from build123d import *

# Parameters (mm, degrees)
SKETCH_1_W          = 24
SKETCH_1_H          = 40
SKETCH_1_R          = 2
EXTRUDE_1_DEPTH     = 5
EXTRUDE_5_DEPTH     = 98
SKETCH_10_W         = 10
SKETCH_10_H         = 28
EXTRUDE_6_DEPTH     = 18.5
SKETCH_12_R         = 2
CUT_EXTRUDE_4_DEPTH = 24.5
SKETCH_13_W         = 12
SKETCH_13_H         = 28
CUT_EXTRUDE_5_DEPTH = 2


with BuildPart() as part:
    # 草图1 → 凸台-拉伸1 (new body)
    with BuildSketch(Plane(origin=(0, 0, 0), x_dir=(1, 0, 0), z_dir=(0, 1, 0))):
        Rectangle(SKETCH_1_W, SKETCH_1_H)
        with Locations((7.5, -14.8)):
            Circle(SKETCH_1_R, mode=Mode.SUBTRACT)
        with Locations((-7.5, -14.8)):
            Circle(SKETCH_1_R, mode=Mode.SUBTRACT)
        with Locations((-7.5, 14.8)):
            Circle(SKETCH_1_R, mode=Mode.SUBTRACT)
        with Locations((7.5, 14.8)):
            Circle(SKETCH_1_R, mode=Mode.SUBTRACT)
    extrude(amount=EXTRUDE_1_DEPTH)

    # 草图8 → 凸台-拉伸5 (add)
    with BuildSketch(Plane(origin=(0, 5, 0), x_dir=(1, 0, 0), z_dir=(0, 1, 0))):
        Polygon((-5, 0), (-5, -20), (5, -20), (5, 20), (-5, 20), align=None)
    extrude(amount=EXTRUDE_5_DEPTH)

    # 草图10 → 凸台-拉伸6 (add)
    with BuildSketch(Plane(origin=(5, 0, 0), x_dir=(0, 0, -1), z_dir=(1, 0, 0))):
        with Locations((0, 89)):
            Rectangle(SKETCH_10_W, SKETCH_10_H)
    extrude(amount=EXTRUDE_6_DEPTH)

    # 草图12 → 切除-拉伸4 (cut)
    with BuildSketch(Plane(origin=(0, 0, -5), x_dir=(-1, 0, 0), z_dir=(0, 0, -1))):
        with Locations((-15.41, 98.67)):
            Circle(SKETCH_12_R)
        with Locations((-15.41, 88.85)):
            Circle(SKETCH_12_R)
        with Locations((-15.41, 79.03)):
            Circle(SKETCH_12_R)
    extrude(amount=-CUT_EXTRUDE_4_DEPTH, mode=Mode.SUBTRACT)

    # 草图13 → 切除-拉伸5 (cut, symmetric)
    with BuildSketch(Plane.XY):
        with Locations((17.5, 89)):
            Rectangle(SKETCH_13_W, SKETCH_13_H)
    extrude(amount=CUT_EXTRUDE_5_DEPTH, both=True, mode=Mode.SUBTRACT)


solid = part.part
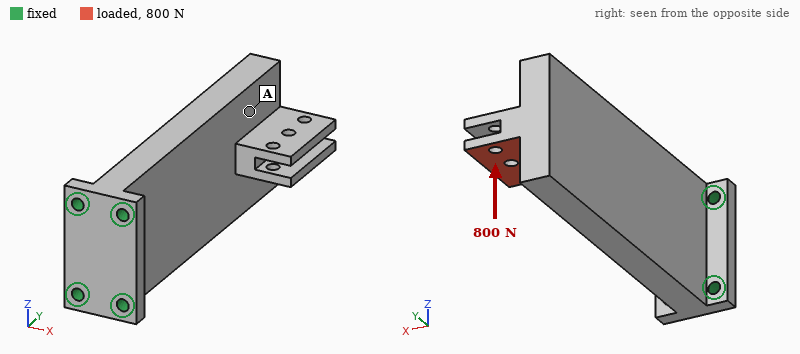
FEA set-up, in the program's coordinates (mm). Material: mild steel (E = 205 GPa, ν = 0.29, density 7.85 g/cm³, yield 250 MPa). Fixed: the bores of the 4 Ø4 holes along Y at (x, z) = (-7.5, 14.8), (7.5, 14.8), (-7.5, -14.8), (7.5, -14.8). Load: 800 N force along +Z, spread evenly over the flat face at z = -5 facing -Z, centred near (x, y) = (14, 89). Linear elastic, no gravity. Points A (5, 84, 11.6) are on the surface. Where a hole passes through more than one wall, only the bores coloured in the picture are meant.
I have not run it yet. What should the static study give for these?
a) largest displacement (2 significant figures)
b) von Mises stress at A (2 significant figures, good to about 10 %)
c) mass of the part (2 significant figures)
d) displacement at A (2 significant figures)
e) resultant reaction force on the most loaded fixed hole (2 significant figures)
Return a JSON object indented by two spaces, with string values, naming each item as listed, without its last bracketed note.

{
  "largest displacement": "70 µm",
  "von Mises stress at A": "12 MPa",
  "mass of the part": "370 g",
  "displacement at A": "28 µm",
  "resultant reaction force on the most loaded fixed hole": "1.5 kN"
}
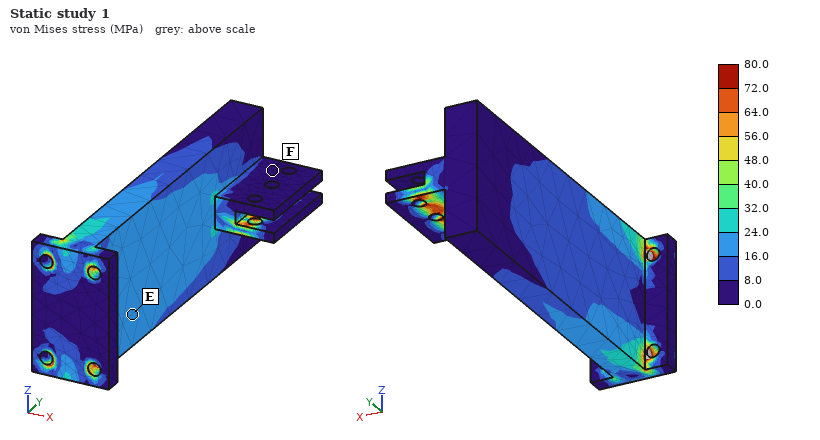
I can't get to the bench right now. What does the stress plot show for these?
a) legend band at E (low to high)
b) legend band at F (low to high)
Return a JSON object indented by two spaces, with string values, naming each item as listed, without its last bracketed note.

{
  "legend band at E": "16.0 to 24.0 MPa",
  "legend band at F": "0.0 to 8.0 MPa"
}
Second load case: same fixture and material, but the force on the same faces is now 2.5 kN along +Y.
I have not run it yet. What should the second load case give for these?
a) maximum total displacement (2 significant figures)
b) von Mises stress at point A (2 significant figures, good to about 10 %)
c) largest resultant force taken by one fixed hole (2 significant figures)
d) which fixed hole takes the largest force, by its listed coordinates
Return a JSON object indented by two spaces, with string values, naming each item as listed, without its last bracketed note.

{
  "maximum total displacement": "0.29 mm",
  "von Mises stress at point A": "26 MPa",
  "largest resultant force taken by one fixed hole": "2.2 kN",
  "which fixed hole takes the largest force, by its listed coordinates": "(7.5, -14.8)"
}
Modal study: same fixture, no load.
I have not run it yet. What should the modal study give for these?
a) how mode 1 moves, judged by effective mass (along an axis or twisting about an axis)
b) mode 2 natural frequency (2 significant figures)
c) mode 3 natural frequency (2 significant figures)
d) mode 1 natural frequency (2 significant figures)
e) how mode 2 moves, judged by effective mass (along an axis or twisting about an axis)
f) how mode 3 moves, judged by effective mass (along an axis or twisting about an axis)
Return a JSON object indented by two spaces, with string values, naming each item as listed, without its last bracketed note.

{
  "how mode 1 moves, judged by effective mass": "along X",
  "mode 2 natural frequency": "2300 Hz",
  "mode 3 natural frequency": "3500 Hz",
  "mode 1 natural frequency": "690 Hz",
  "how mode 2 moves, judged by effective mass": "along Z",
  "how mode 3 moves, judged by effective mass": "twisting about Y"
}
